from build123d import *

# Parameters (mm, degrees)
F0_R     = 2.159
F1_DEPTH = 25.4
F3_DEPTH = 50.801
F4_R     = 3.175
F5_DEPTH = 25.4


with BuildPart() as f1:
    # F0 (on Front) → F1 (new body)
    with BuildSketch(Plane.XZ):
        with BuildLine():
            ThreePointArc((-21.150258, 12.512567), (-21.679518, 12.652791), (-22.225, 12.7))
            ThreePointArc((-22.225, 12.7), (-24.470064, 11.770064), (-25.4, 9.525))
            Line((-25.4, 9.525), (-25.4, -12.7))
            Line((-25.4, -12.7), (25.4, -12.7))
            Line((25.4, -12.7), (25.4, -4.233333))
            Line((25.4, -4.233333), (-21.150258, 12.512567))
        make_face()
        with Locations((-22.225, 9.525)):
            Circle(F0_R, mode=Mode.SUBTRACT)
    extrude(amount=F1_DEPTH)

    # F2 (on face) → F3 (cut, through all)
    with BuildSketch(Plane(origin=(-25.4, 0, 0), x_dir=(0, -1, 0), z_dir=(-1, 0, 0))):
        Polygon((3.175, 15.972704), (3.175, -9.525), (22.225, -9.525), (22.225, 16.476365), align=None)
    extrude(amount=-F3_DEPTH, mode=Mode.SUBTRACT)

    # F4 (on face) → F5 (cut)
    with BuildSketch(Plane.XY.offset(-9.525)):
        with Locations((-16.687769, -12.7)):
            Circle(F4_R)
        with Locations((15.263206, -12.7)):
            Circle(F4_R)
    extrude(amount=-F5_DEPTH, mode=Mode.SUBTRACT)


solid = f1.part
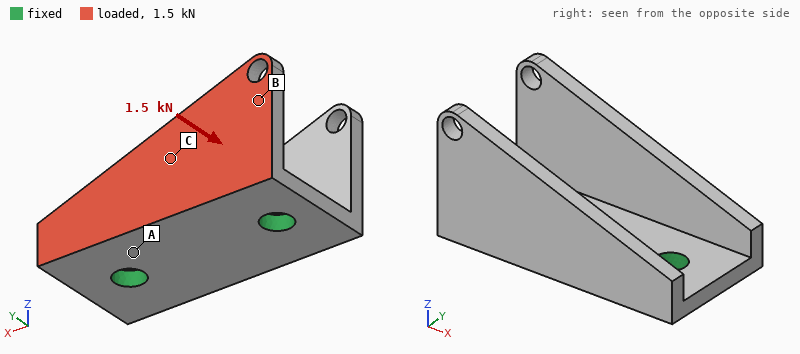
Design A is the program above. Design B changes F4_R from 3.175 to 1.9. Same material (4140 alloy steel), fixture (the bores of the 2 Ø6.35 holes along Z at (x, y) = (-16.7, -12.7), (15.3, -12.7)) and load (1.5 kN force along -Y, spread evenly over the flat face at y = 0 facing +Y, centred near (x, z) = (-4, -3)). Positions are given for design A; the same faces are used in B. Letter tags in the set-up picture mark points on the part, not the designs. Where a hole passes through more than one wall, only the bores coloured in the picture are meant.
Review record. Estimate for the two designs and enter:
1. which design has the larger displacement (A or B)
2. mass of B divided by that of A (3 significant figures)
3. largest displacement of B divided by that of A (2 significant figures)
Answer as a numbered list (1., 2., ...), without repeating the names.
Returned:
1. B
2. 1.02
3. 1.1
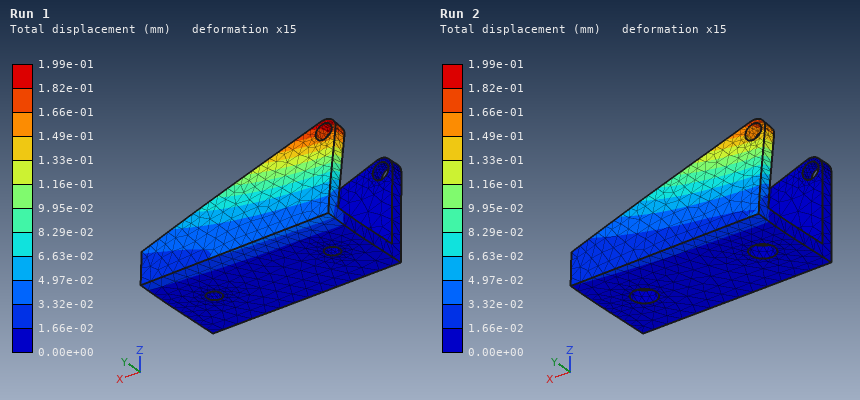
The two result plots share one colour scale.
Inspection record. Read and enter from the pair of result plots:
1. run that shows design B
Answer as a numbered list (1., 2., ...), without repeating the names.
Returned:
1. Run 1
